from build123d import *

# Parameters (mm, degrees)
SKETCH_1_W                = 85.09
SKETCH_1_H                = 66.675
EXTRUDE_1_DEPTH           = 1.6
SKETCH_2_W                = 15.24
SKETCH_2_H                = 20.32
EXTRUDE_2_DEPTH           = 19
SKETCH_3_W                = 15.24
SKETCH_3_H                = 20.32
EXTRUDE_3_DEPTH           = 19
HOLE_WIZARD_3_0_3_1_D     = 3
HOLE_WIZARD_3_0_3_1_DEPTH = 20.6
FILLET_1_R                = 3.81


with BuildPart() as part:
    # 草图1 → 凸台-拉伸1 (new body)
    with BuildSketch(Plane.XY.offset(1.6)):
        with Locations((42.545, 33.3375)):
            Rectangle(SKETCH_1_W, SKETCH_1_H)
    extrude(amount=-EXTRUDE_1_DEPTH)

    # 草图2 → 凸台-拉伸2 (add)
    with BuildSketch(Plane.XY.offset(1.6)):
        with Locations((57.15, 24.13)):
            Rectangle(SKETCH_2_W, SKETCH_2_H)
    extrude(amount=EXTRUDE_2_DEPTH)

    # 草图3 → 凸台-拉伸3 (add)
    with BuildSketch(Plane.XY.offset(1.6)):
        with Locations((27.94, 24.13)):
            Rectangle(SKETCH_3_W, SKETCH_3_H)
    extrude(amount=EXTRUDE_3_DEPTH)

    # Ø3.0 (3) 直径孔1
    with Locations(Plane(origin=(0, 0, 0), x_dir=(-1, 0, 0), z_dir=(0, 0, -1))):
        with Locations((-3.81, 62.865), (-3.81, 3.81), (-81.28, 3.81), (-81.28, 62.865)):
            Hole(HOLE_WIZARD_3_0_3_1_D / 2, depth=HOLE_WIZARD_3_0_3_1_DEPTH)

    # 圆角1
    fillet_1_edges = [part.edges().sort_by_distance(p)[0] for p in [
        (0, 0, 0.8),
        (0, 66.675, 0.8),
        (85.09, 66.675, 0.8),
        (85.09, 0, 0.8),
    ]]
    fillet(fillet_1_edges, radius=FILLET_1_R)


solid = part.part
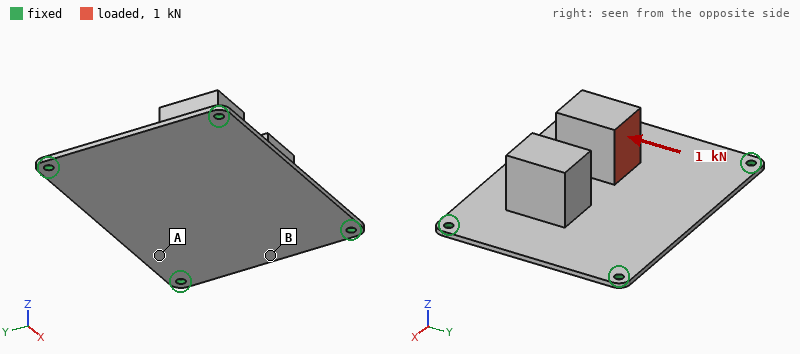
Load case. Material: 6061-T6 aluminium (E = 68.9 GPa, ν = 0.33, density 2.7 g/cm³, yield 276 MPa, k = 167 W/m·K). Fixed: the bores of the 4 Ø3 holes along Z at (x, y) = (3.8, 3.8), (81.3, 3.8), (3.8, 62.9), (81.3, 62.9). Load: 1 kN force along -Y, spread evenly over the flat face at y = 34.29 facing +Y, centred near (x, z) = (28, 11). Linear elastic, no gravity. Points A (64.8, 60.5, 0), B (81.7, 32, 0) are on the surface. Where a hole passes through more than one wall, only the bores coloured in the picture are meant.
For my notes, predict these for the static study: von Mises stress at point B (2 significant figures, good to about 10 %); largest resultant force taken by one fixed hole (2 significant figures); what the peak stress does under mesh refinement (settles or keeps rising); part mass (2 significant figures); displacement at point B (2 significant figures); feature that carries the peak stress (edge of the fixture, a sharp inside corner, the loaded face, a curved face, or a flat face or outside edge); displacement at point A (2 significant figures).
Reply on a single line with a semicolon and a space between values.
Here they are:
41 MPa; 410 N; keeps rising; 56 g; 0.11 mm; edge of the fixture; 0.14 mm
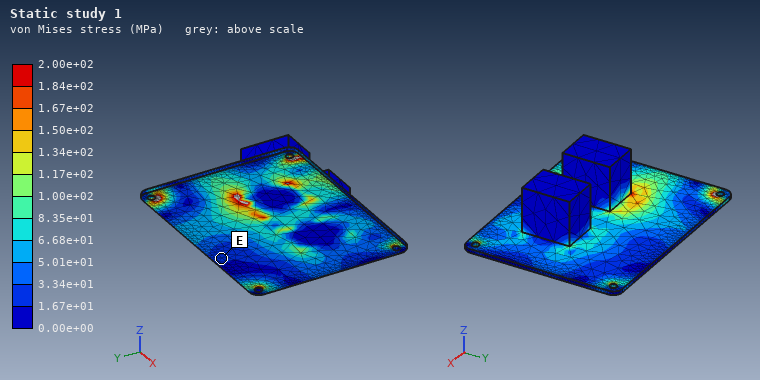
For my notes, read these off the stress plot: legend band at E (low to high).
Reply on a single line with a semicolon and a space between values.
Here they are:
1.67e+01 to 3.34e+01 MPa
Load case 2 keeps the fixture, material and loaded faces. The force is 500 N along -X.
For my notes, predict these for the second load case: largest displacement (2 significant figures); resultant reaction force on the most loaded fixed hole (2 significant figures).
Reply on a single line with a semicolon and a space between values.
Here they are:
0.43 mm; 180 N
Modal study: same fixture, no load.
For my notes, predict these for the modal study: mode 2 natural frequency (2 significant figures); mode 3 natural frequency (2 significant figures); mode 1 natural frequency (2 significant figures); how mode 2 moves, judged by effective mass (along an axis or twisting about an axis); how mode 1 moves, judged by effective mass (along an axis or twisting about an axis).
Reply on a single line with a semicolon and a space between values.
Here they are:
1300 Hz; 1500 Hz; 630 Hz; along Y; along Z
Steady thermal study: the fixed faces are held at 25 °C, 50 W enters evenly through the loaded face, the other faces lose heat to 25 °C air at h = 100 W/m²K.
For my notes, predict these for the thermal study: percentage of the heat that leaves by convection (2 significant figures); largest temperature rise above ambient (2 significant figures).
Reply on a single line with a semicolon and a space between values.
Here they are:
61 %; 60 K
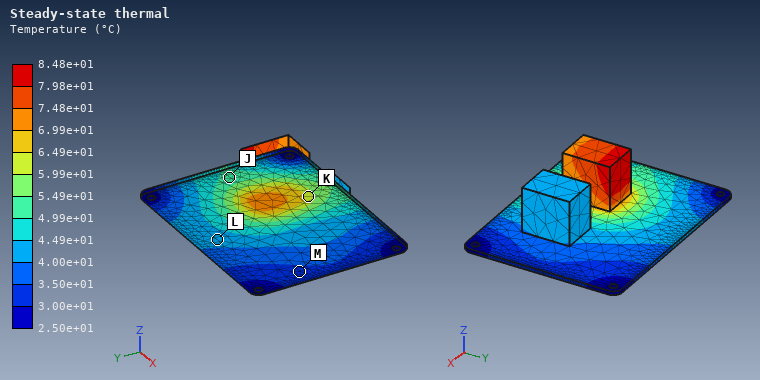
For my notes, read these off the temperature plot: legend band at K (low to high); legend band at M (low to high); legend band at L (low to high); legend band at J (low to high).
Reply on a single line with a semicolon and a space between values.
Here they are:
5.99e+01 to 6.49e+01 °C; 3.00e+01 to 3.50e+01 °C; 4.00e+01 to 4.49e+01 °C; 4.99e+01 to 5.49e+01 °C
